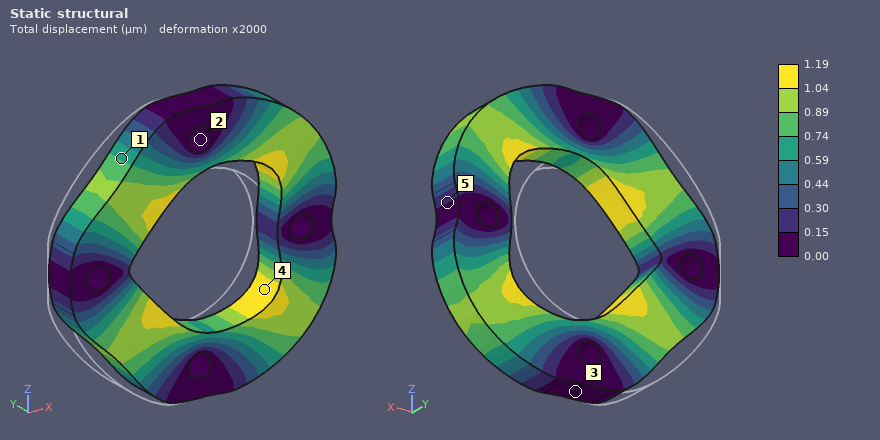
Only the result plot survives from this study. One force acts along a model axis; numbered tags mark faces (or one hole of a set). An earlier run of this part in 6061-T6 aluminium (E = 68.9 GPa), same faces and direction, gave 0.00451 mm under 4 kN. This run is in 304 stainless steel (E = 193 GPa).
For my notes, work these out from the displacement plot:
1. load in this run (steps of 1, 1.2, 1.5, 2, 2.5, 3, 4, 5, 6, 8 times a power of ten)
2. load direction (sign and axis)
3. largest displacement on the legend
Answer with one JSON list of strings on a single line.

["3 kN", "+X", "1.19 µm"]
